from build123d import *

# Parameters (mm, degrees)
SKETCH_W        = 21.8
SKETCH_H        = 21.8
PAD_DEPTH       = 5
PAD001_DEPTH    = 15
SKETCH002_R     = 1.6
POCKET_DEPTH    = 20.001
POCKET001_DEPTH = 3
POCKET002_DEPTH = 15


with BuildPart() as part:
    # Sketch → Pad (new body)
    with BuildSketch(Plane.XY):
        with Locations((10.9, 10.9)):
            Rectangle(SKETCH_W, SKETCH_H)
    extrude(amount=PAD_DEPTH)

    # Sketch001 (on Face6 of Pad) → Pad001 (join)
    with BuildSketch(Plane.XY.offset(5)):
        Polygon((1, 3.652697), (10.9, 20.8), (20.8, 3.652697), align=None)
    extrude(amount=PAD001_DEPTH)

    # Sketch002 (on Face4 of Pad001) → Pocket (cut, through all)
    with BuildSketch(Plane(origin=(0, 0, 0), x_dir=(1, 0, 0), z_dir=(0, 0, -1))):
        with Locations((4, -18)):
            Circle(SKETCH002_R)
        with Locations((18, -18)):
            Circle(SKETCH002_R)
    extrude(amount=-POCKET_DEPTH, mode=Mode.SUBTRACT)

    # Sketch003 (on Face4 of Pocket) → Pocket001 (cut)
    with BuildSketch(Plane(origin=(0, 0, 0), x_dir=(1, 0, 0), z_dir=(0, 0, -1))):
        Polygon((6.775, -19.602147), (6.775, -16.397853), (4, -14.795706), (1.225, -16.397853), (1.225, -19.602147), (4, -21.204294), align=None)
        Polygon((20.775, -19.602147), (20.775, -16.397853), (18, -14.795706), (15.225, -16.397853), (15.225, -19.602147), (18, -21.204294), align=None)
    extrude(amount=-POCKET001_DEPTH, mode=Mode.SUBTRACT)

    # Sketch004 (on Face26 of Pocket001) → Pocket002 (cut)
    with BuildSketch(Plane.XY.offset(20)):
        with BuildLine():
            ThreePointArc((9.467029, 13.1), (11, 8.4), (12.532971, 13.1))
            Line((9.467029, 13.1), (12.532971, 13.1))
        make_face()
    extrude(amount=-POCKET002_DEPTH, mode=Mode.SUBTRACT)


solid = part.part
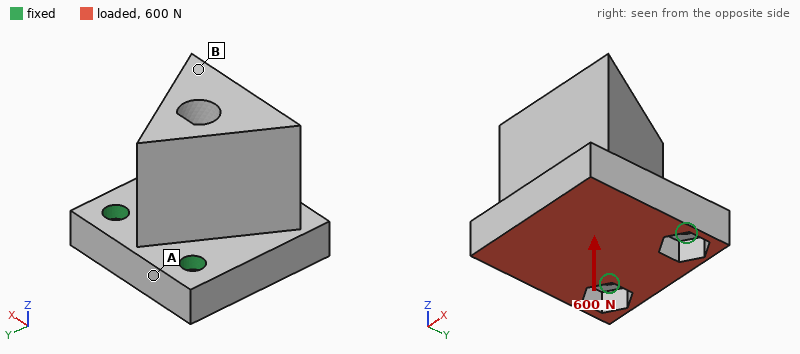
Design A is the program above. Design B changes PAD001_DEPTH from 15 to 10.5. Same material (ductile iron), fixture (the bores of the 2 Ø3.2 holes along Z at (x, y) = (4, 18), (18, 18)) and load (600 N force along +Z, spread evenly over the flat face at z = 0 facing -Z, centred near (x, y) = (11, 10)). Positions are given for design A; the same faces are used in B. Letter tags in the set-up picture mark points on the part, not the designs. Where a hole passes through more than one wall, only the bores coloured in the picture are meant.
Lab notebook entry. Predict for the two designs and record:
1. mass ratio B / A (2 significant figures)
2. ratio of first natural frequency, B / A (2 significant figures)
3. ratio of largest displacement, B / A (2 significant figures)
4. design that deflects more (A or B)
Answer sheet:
0.85
1.2
0.87
A
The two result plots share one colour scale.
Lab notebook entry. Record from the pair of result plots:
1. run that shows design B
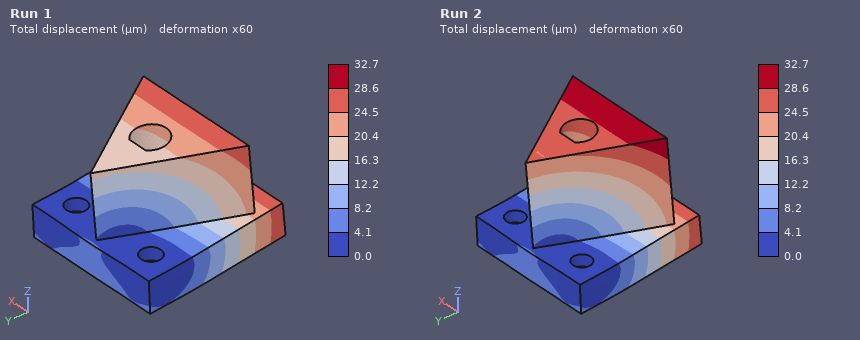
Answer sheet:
Run 1
